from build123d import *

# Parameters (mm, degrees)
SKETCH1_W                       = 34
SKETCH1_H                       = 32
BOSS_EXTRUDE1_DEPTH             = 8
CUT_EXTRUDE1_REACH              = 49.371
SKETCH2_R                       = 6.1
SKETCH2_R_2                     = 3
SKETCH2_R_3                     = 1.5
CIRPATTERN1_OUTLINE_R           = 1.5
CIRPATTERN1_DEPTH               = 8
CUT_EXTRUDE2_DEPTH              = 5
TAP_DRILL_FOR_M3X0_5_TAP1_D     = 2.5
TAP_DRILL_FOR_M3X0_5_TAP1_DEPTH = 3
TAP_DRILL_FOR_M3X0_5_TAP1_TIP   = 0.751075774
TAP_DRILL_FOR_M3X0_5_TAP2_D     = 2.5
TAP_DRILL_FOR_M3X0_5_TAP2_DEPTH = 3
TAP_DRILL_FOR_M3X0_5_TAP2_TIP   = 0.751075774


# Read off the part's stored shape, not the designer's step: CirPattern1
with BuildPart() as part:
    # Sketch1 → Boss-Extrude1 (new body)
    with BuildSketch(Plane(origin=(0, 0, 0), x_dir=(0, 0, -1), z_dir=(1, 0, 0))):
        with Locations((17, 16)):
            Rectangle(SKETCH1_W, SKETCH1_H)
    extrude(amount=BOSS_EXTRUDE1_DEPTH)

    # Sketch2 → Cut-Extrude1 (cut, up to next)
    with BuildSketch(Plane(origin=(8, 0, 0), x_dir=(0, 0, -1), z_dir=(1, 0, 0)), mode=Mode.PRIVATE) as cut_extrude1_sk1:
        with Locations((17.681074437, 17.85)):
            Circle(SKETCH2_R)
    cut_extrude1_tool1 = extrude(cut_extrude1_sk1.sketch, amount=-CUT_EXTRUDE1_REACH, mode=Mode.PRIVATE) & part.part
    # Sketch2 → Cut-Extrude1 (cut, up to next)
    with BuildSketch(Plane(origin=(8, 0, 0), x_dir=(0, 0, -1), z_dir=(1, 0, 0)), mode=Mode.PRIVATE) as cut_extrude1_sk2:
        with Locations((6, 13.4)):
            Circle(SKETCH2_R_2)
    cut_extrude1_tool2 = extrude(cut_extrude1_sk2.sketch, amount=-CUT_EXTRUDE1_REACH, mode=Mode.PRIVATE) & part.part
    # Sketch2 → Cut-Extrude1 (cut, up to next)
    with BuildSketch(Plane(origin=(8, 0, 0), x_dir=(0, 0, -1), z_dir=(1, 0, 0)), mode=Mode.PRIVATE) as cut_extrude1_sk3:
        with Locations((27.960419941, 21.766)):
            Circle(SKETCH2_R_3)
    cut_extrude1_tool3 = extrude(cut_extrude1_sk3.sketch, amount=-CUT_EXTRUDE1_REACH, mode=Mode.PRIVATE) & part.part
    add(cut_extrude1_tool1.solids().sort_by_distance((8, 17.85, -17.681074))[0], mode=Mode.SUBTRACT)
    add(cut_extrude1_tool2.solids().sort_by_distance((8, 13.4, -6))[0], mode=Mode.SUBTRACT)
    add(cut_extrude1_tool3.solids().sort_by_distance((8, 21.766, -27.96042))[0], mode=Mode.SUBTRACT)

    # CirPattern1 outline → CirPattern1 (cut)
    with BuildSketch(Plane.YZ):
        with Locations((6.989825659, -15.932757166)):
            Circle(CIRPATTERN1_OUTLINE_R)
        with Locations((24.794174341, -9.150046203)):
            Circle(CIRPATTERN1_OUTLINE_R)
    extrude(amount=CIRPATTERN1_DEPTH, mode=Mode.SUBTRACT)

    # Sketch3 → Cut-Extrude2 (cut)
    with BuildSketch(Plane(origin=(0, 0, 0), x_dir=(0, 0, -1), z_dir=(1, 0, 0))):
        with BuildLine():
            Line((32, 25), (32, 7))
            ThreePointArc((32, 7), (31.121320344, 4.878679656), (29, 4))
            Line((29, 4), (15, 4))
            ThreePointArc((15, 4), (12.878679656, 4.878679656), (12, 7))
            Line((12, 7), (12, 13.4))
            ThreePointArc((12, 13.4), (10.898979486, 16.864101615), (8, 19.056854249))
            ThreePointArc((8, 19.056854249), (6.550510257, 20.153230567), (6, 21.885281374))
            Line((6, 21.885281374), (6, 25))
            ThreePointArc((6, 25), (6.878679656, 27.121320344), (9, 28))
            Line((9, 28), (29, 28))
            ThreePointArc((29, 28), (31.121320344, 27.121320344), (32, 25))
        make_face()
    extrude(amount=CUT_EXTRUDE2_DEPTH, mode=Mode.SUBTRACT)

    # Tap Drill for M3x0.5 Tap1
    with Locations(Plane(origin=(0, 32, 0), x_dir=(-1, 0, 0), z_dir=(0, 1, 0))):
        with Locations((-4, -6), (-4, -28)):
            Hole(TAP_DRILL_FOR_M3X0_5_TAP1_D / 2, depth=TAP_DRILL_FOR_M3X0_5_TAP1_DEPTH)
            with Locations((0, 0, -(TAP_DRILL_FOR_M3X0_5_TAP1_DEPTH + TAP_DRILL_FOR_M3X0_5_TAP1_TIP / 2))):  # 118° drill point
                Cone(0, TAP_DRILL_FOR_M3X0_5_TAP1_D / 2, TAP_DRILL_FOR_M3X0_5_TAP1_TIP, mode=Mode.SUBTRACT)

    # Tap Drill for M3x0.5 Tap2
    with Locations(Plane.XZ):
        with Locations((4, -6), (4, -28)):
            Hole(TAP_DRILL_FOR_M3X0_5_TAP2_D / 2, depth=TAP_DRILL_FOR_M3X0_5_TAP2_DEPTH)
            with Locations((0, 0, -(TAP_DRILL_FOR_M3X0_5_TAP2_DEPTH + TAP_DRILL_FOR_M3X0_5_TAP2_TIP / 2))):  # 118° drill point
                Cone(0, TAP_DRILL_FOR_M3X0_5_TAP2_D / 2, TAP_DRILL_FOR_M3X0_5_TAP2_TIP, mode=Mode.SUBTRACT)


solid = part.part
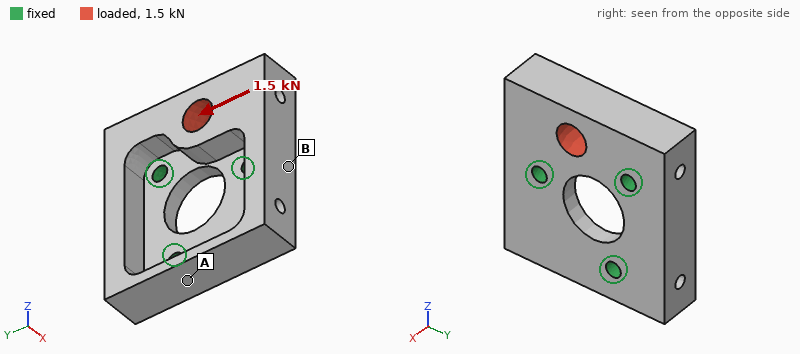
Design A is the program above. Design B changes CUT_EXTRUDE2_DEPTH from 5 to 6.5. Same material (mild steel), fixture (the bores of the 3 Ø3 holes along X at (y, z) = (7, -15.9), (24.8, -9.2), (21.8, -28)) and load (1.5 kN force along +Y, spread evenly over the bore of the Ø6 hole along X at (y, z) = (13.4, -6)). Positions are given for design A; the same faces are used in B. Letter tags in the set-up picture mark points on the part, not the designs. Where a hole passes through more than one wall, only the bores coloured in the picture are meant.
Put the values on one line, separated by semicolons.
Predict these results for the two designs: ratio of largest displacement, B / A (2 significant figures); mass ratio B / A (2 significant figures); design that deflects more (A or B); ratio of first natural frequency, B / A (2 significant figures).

2.3; 0.89; B; 0.70
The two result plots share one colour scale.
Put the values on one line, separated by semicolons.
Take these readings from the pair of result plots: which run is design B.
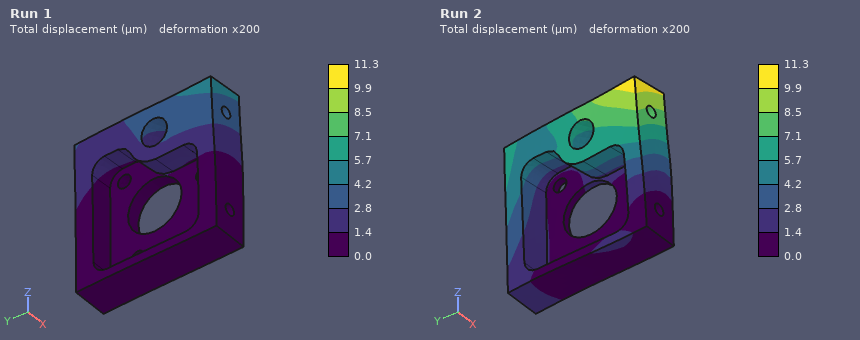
Run 2
